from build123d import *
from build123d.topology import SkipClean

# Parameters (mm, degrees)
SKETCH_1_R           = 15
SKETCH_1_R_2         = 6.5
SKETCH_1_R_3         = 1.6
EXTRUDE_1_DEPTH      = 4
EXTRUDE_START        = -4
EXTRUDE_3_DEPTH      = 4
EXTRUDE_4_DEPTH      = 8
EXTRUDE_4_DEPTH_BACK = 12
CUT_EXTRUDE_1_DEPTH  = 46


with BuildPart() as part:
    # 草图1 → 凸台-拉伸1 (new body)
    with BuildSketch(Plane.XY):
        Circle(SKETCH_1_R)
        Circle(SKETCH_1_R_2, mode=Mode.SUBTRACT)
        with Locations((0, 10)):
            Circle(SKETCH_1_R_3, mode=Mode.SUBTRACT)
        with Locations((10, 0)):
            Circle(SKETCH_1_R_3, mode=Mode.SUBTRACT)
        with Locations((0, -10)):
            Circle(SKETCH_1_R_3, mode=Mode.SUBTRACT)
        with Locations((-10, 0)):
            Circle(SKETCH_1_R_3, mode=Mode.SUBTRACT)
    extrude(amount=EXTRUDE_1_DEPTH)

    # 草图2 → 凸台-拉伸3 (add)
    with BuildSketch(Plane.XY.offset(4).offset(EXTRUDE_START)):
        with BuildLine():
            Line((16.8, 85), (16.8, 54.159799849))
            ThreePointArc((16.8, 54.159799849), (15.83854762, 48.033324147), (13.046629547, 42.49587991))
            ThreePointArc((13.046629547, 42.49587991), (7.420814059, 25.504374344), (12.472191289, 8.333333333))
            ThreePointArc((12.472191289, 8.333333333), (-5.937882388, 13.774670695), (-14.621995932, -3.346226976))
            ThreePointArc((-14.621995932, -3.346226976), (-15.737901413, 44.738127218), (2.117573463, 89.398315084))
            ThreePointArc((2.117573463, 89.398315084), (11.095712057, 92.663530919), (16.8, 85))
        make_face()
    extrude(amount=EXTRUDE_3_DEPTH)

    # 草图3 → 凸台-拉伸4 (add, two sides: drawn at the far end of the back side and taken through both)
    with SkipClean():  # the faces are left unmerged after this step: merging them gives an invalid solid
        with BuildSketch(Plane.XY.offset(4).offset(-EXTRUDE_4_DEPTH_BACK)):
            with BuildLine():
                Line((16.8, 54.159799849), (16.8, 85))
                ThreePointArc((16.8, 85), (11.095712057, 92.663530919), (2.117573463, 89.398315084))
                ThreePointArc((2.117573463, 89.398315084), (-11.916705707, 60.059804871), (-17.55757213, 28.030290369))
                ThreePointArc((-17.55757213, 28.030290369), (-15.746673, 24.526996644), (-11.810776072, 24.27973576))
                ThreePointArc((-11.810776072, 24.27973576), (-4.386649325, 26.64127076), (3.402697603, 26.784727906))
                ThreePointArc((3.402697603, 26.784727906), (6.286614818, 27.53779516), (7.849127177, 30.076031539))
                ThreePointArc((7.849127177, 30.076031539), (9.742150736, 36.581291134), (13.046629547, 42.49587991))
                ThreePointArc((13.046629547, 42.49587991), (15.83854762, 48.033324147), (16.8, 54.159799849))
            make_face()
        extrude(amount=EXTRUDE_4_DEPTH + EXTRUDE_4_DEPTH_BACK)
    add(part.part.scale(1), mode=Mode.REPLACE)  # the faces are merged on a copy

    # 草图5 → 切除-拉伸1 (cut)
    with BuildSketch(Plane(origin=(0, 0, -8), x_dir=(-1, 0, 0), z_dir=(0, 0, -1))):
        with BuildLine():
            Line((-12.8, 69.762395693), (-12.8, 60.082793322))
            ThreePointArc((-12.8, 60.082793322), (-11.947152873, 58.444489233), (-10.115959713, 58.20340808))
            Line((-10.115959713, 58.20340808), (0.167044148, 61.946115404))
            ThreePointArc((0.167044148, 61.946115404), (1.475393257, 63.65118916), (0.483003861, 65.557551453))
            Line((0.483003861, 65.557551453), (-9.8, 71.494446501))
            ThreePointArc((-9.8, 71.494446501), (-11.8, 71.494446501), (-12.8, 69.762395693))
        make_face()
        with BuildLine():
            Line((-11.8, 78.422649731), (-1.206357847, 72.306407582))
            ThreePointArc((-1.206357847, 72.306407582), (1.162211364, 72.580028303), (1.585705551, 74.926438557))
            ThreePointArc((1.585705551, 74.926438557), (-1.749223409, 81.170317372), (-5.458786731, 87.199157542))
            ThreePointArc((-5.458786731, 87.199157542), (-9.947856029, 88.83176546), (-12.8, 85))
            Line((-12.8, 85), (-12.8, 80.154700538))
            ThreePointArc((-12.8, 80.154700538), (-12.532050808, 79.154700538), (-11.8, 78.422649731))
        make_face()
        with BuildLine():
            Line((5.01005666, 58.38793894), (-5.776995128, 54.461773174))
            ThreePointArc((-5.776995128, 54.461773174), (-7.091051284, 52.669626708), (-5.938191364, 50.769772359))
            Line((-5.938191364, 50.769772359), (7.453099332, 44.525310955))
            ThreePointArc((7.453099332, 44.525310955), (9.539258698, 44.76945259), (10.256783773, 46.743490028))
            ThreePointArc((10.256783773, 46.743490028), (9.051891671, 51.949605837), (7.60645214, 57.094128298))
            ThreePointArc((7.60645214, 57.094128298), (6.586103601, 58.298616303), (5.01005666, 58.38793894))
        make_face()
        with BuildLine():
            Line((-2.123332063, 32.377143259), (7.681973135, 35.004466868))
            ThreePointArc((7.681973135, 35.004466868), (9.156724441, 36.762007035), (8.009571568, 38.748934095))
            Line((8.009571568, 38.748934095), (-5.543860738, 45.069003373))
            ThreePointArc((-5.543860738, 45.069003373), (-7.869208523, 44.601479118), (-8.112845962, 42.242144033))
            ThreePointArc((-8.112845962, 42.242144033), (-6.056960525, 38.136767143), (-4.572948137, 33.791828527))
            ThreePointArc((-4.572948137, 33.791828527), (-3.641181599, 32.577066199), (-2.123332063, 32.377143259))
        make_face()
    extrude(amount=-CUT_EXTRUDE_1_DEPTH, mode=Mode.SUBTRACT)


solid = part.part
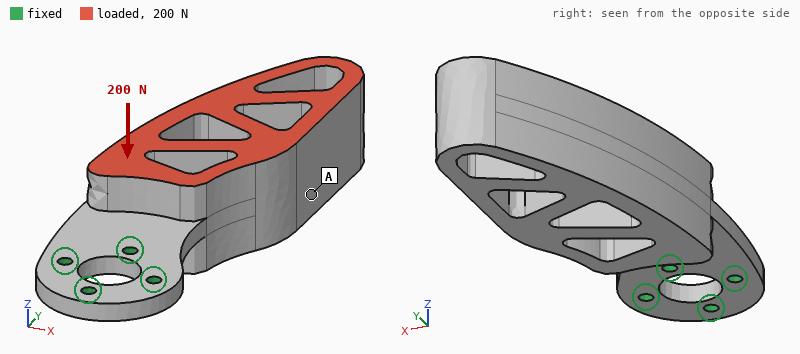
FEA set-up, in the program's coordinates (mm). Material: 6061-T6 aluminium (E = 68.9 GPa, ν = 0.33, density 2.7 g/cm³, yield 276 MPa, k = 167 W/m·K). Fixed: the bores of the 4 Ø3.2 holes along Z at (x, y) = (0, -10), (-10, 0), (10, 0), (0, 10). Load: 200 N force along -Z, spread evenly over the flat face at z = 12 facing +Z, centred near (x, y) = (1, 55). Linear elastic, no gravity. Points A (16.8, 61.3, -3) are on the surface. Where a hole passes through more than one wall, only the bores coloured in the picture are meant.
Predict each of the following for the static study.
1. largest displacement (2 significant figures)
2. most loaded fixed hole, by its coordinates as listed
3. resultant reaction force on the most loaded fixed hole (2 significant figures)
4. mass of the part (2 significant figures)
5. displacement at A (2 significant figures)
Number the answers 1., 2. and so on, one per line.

1. 1.0 mm
2. (0, 10)
3. 600 N
4. 70 g
5. 0.57 mm
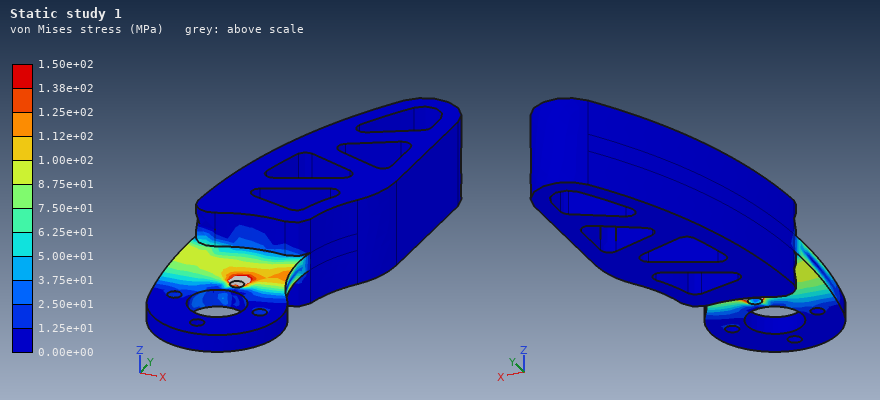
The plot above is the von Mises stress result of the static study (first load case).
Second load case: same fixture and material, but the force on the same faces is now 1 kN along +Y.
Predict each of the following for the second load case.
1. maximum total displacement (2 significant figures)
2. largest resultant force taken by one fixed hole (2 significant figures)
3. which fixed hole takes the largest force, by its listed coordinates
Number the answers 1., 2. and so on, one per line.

1. 1.4 mm
2. 810 N
3. (0, 10)
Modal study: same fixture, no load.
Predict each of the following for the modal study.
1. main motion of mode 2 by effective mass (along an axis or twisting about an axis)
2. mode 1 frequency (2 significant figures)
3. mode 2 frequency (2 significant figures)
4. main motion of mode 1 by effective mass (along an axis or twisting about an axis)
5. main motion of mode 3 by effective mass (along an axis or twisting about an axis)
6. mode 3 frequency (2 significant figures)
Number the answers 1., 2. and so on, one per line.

1. along X
2. 370 Hz
3. 1600 Hz
4. along Z
5. twisting about Y
6. 1900 Hz
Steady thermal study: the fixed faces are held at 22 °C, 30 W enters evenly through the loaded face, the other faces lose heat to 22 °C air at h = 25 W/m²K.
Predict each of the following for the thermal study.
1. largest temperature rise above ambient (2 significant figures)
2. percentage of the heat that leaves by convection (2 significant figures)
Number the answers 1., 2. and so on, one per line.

1. 42 K
2. 26 %
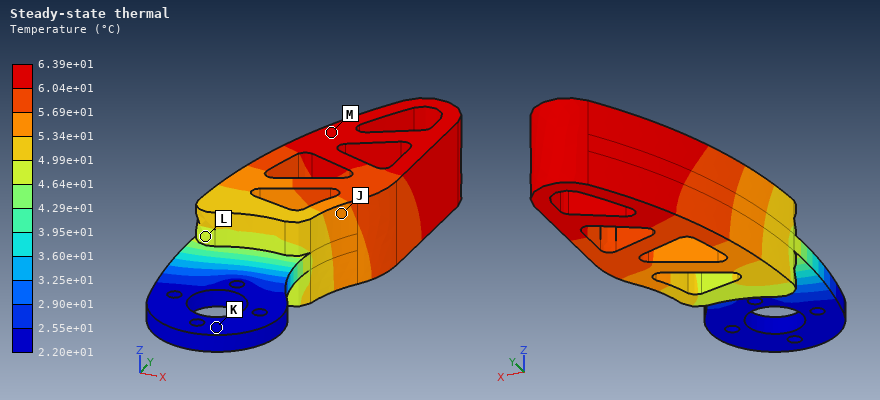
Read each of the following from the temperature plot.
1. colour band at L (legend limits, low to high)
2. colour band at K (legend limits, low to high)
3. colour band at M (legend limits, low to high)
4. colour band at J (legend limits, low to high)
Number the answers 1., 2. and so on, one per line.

1. 4.64e+01 to 4.99e+01 °C
2. 2.20e+01 to 2.55e+01 °C
3. 6.04e+01 to 6.39e+01 °C
4. 5.34e+01 to 5.69e+01 °C
